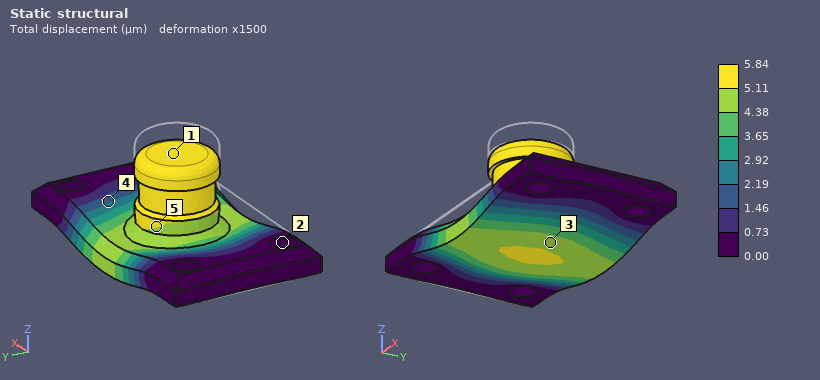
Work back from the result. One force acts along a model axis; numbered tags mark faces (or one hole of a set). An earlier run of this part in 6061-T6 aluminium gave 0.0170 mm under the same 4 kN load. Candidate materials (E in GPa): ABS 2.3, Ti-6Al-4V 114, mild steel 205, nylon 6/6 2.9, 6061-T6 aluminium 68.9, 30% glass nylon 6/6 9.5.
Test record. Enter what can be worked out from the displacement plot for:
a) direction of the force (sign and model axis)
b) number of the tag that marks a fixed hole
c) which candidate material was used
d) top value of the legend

-Z
2
mild steel
5.84 µm
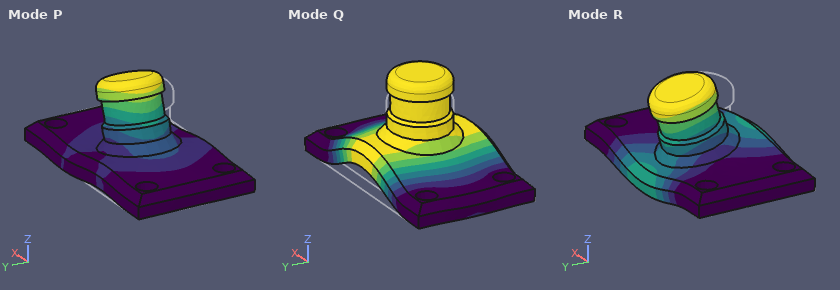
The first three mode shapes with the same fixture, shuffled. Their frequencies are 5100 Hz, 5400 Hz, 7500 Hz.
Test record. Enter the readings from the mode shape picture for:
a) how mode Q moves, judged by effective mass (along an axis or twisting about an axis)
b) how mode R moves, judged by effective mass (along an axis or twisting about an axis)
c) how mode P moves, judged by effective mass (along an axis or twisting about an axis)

along Z
along Y
along X
